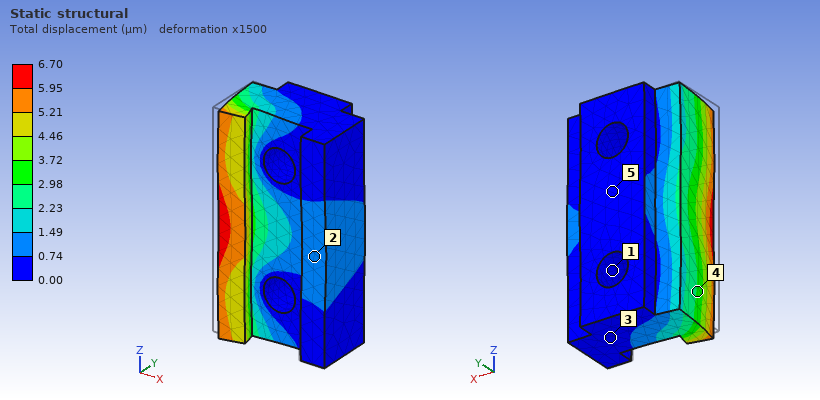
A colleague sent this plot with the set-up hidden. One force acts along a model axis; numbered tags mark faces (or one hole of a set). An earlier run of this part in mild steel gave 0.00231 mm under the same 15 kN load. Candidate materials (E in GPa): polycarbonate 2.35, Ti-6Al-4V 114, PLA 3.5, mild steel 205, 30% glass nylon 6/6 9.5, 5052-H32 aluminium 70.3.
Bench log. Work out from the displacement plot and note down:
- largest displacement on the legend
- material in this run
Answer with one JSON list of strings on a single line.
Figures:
["6.70 µm", "5052-H32 aluminium"]
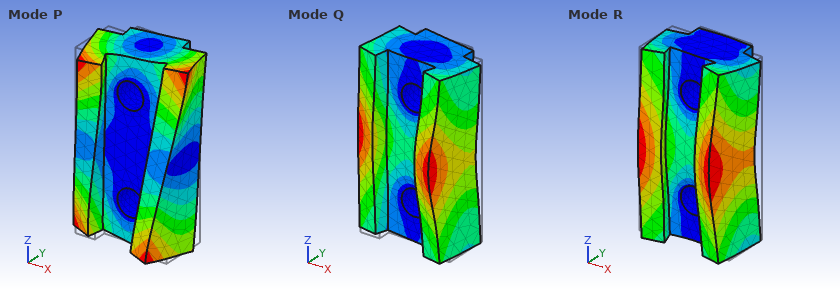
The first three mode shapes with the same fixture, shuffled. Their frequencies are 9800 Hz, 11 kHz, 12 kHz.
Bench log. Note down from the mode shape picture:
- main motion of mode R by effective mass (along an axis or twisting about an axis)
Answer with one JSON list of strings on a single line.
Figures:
["along Y"]
